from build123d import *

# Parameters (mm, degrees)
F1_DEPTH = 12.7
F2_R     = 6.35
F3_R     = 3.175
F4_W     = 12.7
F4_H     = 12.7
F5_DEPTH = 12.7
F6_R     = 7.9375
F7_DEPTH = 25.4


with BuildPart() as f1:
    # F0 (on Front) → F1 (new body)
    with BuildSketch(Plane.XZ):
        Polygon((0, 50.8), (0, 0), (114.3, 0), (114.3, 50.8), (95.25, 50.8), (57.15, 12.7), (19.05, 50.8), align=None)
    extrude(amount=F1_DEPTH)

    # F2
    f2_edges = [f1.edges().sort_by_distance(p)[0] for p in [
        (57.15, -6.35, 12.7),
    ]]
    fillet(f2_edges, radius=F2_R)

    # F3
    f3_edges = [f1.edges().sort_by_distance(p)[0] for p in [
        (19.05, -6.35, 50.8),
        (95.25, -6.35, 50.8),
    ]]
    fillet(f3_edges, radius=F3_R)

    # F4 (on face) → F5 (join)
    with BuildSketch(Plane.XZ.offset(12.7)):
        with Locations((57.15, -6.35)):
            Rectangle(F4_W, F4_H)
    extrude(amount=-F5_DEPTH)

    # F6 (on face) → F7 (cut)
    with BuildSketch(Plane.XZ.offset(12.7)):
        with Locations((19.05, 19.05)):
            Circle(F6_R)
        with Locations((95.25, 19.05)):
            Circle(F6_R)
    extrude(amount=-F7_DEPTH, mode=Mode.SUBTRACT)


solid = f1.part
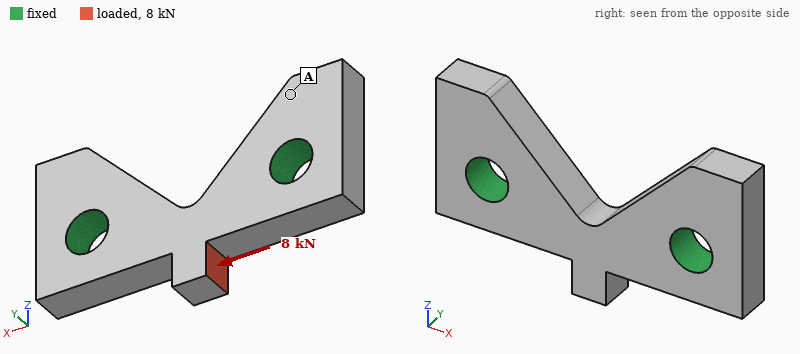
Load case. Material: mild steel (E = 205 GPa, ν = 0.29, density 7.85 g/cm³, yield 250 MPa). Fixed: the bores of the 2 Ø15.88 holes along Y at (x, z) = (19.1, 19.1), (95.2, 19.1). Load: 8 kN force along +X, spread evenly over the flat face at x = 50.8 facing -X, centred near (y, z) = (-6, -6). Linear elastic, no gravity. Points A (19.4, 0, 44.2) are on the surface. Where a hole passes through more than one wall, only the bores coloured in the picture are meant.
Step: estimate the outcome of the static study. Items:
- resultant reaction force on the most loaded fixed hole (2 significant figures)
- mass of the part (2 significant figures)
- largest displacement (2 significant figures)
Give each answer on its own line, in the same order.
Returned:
5.2 kN
410 g
26 µm
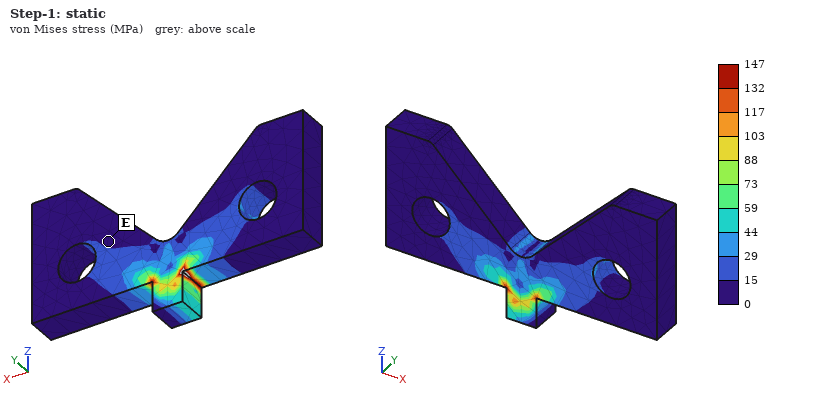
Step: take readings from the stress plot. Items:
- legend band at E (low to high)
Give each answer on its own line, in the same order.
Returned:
0 to 15 MPa
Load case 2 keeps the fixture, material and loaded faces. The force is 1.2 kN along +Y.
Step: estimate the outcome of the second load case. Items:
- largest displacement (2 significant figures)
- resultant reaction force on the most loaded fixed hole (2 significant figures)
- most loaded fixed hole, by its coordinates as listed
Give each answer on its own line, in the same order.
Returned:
18 µm
760 N
(19.1, 19.1)
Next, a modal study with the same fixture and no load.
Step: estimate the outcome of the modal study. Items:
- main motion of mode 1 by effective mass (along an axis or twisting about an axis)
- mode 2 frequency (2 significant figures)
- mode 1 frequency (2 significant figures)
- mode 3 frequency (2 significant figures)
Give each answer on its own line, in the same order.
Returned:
along Y
14 kHz
9500 Hz
14 kHz
